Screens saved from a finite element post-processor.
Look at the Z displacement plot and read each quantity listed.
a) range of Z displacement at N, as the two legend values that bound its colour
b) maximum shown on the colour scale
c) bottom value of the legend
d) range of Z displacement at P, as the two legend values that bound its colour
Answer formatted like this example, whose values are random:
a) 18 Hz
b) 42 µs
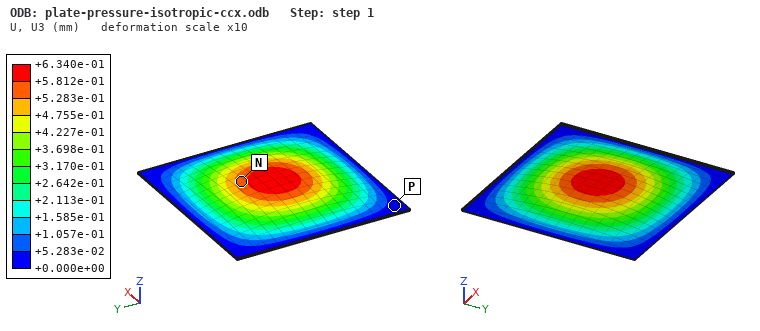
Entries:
a) +5.283e-01 to +5.812e-01 mm
b) +6.340e-01 mm
c) +0.000e+00 mm
d) +0.000e+00 to +5.283e-02 mm
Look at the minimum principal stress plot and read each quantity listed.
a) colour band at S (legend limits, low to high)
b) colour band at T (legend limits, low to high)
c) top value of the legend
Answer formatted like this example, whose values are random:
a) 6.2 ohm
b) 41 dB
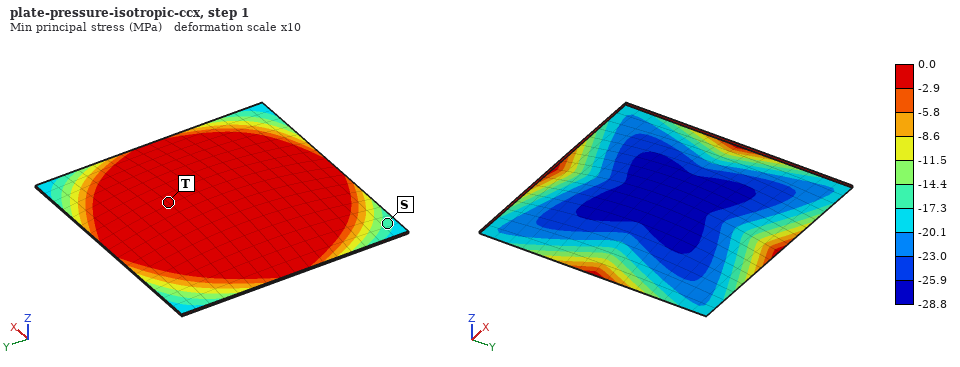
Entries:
a) -17.3 to -14.4 MPa
b) -2.9 to 0.0 MPa
c) 0.0 MPa
